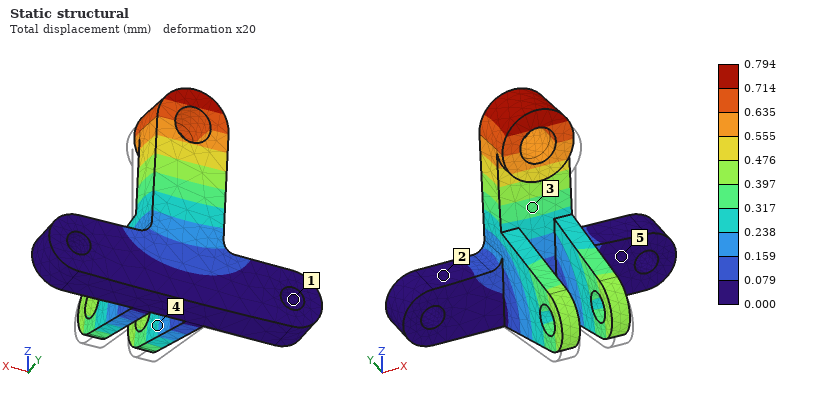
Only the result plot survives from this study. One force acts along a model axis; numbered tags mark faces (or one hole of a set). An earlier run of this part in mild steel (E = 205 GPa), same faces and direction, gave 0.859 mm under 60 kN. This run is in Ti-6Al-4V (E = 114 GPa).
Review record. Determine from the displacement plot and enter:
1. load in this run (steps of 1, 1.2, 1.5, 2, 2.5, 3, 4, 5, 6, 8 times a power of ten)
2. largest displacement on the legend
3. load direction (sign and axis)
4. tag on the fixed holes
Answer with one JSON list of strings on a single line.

["30 kN", "0.794 mm", "+Y", "1"]
